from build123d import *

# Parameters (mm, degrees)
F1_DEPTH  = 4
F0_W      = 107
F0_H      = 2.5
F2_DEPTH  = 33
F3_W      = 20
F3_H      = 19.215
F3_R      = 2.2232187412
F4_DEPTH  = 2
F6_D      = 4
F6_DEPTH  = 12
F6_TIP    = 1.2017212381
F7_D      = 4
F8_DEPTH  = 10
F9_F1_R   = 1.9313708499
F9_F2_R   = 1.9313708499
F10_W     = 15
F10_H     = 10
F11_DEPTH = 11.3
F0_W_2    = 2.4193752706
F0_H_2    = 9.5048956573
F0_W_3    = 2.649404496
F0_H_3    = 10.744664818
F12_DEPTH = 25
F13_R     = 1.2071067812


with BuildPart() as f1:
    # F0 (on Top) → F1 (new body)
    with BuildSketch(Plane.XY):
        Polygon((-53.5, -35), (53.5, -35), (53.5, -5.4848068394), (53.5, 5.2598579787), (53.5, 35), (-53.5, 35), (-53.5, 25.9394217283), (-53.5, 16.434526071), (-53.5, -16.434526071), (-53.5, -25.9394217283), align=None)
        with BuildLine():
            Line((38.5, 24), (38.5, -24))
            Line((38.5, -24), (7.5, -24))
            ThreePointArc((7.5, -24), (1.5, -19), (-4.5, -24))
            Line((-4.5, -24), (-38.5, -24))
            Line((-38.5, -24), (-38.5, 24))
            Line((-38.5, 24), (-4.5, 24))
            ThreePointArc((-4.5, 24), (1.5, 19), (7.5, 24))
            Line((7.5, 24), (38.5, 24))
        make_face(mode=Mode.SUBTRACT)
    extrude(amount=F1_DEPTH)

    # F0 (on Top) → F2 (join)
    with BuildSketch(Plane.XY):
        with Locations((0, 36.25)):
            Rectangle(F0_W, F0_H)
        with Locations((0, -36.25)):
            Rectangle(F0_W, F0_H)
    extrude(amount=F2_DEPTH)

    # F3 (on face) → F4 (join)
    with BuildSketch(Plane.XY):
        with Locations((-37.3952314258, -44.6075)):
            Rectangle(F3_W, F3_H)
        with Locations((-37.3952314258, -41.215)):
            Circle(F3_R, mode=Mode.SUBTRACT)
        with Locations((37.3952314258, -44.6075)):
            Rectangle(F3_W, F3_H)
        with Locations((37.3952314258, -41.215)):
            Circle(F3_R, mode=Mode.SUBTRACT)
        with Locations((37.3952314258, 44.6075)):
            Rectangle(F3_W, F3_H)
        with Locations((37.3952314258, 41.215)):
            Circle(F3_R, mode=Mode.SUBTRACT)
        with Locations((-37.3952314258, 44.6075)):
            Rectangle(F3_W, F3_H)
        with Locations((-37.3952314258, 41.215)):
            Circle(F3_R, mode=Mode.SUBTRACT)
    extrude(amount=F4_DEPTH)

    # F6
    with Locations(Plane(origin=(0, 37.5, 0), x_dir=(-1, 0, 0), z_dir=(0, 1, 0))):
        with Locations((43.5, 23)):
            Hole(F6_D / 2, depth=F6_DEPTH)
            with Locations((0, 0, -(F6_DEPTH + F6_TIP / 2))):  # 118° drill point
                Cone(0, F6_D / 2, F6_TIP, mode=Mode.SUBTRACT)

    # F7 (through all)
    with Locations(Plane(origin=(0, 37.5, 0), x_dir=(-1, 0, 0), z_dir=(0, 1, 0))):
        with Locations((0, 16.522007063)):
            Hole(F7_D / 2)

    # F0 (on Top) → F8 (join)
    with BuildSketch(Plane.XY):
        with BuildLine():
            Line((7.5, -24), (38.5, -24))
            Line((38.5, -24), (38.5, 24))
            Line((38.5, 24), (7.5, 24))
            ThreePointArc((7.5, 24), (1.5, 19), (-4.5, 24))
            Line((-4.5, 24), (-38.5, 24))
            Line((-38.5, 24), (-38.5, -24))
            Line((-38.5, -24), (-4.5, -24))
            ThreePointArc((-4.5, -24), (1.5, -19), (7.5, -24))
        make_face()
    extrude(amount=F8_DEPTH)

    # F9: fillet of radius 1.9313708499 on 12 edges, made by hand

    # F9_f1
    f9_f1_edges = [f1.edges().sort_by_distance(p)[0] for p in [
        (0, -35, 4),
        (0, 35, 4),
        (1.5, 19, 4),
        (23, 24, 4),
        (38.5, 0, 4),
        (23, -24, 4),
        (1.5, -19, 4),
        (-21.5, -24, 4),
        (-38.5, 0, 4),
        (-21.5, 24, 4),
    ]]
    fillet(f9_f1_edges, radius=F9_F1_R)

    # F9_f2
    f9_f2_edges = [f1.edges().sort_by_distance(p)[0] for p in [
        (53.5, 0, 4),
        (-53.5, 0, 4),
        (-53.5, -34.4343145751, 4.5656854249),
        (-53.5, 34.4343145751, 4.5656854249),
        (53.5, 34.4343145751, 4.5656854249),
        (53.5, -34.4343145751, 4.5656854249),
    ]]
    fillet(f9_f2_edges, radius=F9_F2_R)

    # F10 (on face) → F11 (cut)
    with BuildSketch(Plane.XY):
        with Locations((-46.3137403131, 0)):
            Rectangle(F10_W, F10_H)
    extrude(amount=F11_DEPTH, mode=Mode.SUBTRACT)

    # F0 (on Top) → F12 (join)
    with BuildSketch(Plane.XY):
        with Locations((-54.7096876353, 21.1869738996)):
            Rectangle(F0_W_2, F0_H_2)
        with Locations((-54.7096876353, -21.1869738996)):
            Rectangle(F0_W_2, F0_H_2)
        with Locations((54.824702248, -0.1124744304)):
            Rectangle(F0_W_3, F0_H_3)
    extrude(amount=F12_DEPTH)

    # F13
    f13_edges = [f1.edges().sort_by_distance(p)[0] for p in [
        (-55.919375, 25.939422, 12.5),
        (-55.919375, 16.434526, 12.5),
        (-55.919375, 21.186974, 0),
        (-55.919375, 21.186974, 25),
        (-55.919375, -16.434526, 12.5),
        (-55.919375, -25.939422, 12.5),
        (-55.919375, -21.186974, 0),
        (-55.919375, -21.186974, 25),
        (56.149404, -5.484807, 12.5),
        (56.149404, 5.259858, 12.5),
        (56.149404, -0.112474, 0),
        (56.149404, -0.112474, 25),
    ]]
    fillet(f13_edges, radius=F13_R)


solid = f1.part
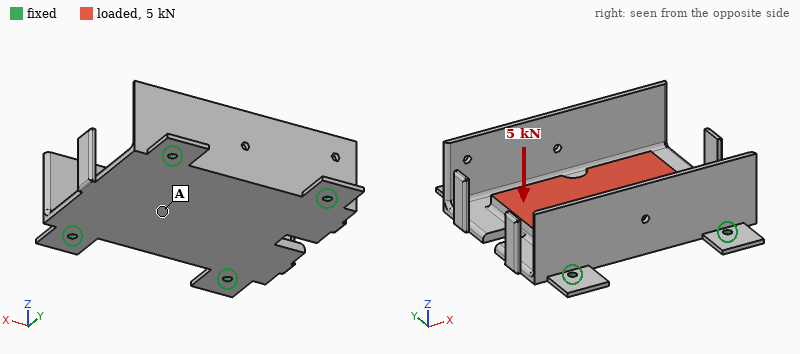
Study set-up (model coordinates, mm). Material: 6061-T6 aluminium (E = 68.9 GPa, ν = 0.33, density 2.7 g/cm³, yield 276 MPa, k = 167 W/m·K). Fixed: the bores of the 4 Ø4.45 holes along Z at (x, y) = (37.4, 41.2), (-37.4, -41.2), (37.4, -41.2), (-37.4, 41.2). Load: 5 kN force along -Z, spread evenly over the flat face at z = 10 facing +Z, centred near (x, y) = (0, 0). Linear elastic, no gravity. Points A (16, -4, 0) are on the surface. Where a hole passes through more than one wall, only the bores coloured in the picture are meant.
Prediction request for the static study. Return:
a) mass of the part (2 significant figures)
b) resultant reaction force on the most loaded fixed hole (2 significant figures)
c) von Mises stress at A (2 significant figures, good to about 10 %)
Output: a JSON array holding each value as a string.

["200 g", "2.4 kN", "29 MPa"]
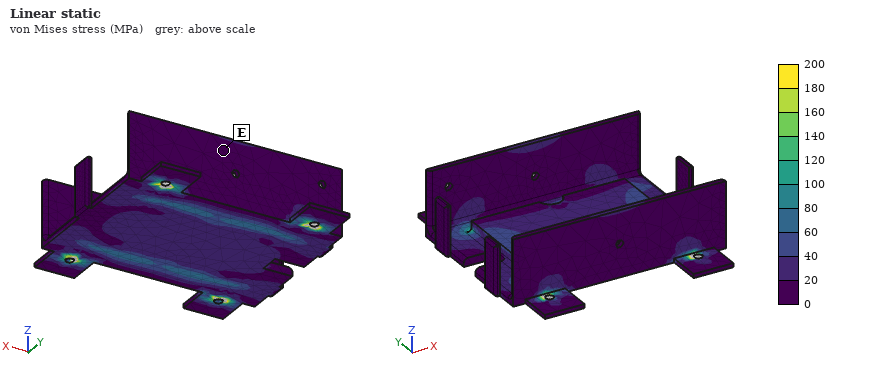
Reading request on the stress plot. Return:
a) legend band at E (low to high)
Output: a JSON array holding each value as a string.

["0 to 20 MPa"]
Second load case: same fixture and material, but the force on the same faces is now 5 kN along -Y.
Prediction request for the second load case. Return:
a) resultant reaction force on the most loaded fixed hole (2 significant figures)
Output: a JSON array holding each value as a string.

["1.3 kN"]
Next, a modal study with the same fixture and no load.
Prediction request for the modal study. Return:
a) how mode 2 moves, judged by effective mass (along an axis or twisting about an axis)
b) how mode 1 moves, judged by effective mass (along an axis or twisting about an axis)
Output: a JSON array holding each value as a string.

["along Y", "along Z"]
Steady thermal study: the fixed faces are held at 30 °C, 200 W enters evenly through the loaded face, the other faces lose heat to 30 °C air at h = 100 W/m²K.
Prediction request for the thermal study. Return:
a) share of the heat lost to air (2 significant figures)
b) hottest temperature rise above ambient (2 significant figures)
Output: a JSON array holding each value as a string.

["49 %", "56 K"]
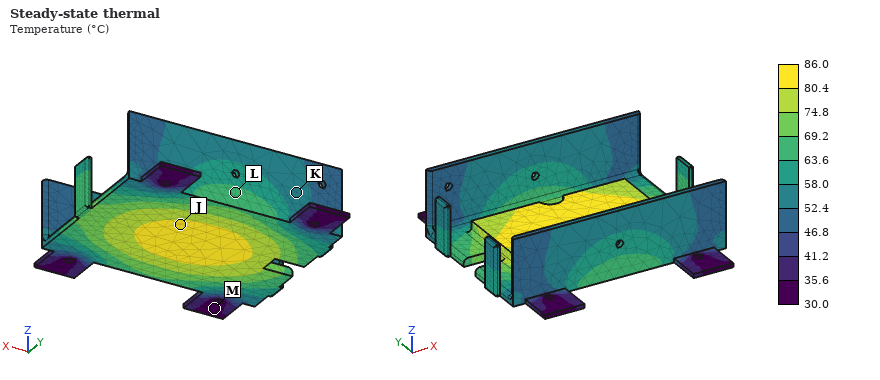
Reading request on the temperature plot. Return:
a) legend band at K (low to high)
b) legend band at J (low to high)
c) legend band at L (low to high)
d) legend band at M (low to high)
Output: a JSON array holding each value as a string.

["52.4 to 58.0 °C", "80.4 to 86.0 °C", "63.6 to 69.2 °C", "30.0 to 35.6 °C"]
